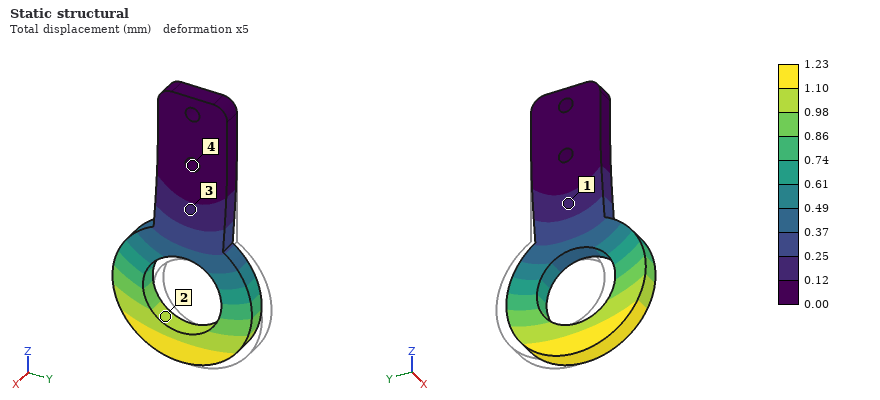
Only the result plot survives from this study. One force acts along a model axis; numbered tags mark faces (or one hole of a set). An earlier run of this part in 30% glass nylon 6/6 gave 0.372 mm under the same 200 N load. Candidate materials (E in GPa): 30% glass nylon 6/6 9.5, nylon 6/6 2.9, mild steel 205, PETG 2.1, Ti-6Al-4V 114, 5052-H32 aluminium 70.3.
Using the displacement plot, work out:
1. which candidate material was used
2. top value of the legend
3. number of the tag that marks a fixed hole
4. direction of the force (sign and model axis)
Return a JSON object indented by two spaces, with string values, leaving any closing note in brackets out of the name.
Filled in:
{
  "which candidate material was used": "nylon 6/6",
  "top value of the legend": "1.23 mm",
  "number of the tag that marks a fixed hole": "4",
  "direction of the force": "-Y"
}
